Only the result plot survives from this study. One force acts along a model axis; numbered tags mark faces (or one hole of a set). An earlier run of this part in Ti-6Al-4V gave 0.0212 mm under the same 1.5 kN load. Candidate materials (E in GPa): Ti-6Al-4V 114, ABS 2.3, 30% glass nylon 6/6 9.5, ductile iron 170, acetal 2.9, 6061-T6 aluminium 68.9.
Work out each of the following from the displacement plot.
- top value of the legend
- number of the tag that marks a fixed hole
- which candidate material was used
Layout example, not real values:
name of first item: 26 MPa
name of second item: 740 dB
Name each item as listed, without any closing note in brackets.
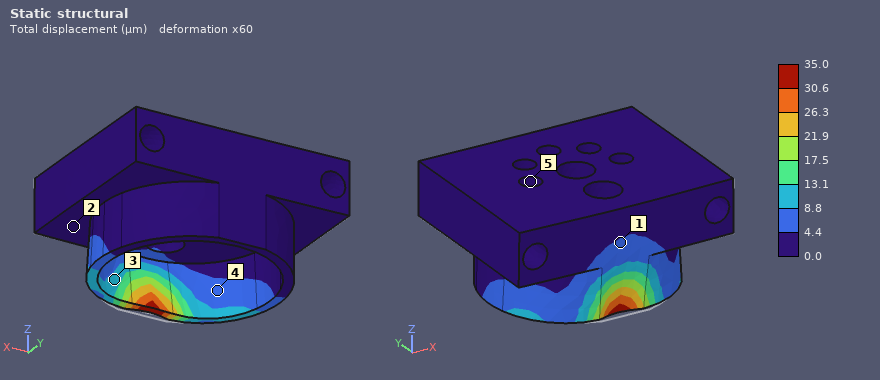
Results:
top value of the legend: 35.0 µm
number of the tag that marks a fixed hole: 5
which candidate material was used: 6061-T6 aluminium
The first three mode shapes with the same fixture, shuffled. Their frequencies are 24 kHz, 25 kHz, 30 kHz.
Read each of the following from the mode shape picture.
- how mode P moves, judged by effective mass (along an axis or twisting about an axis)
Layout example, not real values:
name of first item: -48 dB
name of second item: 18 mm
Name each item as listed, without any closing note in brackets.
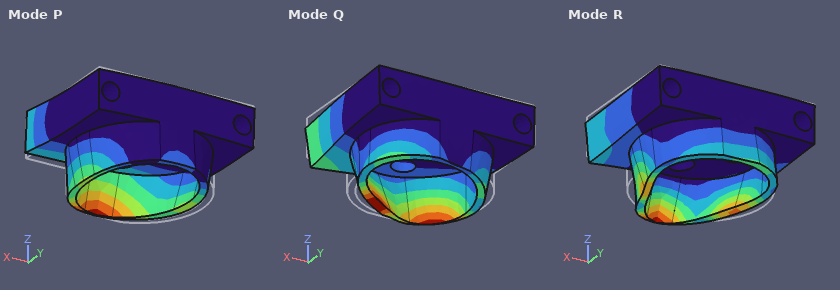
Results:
how mode P moves, judged by effective mass: along Z
